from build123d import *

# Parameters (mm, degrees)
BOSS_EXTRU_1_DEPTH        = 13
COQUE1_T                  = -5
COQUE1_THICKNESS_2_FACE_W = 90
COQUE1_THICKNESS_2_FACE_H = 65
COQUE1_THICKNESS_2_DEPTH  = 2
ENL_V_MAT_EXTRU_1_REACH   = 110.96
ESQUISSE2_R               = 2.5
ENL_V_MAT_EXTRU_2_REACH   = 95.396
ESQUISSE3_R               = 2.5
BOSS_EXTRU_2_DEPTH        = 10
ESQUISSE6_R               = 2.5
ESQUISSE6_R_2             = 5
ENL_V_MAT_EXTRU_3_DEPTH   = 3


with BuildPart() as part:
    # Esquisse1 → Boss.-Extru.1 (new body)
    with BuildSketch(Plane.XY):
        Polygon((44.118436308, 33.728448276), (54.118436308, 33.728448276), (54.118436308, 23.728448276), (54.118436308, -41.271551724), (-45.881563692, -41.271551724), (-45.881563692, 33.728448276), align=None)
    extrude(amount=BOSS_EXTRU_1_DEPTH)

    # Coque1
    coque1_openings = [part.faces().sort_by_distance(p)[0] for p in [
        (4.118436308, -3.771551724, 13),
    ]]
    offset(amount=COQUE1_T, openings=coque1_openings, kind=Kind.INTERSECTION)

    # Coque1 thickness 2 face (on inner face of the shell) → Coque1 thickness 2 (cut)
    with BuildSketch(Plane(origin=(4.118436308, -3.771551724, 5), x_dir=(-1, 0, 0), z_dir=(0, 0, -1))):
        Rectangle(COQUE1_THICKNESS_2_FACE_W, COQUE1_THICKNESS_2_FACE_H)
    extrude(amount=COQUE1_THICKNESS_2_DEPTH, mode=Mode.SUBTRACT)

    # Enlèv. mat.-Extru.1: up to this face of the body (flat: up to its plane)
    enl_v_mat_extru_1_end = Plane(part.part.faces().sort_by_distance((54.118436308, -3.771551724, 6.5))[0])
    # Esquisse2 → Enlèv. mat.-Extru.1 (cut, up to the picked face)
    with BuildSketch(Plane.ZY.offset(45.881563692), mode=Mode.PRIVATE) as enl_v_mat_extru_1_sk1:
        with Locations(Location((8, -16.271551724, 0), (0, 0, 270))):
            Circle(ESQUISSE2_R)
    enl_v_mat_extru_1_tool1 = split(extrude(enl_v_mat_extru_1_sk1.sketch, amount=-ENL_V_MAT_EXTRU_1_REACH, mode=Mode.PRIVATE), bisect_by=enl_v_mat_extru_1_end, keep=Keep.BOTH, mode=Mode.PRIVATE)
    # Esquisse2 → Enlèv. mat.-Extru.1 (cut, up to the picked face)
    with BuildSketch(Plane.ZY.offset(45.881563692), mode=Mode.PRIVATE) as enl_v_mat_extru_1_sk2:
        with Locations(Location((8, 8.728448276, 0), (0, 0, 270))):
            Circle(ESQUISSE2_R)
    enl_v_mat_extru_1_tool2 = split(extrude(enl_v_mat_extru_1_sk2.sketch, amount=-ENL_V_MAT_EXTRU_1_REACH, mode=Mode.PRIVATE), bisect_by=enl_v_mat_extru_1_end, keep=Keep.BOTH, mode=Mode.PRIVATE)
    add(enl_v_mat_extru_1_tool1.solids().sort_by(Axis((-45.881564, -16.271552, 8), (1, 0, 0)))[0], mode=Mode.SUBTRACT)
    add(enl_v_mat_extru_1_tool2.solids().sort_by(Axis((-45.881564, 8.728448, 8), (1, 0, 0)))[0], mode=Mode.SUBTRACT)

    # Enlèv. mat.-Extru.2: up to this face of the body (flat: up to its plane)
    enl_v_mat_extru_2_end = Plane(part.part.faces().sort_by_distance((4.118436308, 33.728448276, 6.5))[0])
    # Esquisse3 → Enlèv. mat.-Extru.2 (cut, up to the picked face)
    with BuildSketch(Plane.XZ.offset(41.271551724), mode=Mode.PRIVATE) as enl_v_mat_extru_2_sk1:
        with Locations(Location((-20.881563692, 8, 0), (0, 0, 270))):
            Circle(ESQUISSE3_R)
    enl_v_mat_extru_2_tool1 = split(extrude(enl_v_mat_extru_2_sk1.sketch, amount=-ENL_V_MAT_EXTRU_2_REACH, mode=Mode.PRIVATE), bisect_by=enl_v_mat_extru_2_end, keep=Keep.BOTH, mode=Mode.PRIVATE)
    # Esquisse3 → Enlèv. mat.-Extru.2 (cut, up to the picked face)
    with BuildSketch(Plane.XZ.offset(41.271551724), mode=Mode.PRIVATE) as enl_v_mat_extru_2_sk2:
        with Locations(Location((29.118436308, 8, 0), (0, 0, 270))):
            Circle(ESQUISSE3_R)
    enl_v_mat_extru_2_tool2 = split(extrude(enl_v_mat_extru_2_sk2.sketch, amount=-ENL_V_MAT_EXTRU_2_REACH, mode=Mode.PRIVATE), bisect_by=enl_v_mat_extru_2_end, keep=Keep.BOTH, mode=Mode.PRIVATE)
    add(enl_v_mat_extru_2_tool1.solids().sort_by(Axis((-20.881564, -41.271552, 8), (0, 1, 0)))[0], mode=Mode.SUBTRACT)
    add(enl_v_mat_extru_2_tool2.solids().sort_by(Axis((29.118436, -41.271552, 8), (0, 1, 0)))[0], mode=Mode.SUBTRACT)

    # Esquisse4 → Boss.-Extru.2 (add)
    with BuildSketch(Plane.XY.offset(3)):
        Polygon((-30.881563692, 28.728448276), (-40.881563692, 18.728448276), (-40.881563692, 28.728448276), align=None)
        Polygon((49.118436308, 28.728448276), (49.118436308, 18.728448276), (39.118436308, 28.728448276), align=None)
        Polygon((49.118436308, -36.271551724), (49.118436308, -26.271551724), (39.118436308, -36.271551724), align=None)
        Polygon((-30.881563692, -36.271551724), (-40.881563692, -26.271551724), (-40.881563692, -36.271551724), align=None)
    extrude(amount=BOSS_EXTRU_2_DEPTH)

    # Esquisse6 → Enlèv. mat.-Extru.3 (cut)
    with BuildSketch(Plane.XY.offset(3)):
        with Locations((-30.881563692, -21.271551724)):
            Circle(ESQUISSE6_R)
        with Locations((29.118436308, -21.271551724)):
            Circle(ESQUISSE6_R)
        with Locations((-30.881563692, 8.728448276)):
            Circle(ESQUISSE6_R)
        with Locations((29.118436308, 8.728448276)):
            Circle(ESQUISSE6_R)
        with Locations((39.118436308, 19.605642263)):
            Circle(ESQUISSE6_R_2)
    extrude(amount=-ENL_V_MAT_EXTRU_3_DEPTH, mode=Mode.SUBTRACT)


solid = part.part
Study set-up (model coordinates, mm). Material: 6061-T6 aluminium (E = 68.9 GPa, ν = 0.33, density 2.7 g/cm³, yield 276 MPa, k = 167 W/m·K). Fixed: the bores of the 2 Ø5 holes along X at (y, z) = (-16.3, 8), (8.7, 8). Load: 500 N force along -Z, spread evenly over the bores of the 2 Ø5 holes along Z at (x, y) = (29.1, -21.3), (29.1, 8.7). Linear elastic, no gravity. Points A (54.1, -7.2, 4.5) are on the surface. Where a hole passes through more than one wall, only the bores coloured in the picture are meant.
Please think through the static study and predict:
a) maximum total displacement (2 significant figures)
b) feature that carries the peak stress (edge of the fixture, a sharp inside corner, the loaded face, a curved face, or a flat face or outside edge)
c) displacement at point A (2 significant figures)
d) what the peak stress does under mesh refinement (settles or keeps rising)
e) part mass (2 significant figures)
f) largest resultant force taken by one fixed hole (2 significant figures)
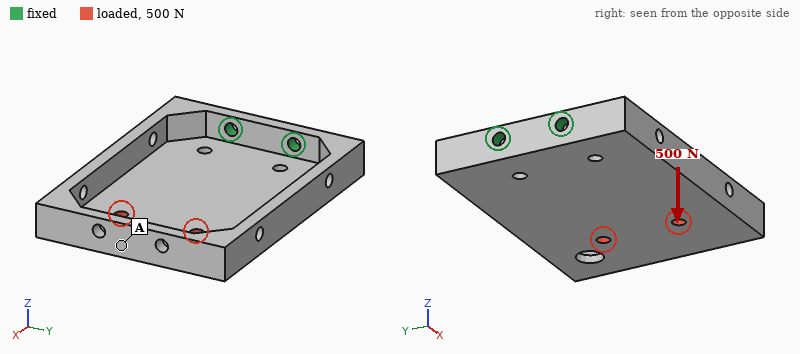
1.4 mm
edge of the fixture
1.4 mm
keeps rising
110 g
560 N
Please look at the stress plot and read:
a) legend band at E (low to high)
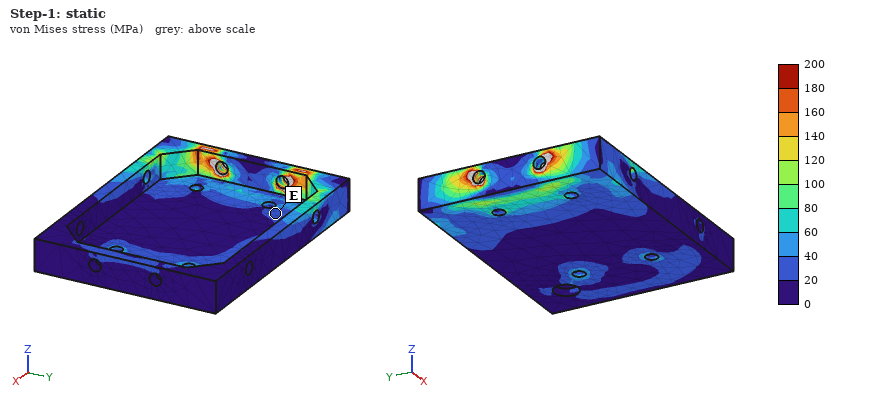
20 to 40 MPa
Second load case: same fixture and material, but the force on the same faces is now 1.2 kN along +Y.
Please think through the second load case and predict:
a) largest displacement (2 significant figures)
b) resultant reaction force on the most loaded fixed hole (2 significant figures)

0.36 mm
2.9 kN
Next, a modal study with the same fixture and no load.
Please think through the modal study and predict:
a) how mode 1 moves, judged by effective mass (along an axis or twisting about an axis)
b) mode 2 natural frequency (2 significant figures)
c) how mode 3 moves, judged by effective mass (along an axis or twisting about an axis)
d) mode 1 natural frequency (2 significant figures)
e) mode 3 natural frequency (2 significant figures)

along Z
860 Hz
along Y
430 Hz
1600 Hz
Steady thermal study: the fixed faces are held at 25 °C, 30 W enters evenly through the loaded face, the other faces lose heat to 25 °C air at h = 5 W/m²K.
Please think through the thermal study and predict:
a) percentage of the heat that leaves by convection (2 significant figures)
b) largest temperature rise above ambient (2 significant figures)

11 %
52 K
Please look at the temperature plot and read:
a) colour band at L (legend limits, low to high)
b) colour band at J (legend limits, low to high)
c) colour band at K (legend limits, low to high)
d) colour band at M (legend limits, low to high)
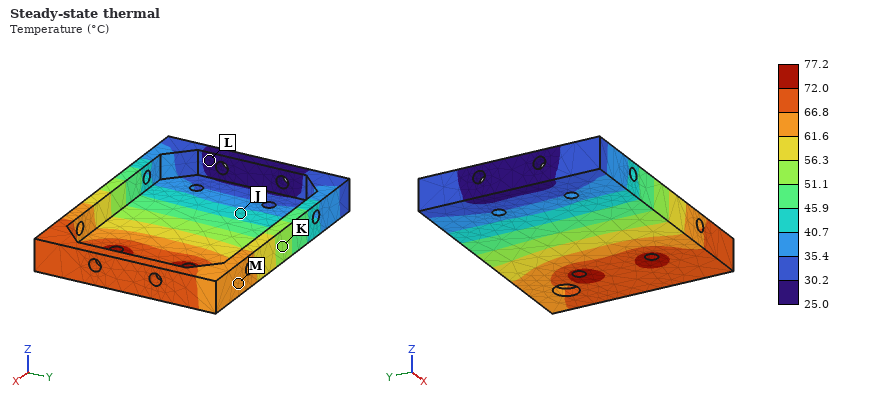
25.0 to 30.2 °C
40.7 to 45.9 °C
51.1 to 56.3 °C
61.6 to 66.8 °C
